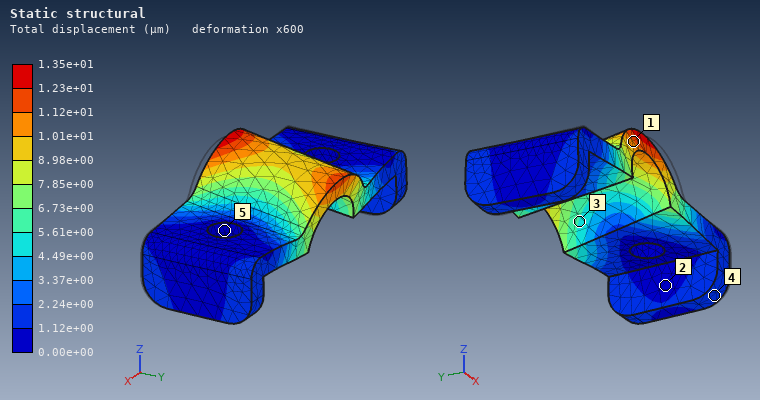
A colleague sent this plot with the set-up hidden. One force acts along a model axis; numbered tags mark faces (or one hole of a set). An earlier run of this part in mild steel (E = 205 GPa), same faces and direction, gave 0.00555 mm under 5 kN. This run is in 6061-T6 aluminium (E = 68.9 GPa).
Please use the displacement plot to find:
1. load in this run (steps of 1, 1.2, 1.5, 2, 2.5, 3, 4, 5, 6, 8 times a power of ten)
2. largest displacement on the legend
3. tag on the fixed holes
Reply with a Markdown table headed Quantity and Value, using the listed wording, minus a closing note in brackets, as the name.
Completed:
| Quantity | Value |
|---|---|
| load in this run | 4 kN |
| largest displacement on the legend | 1.35e+01 µm |
| tag on the fixed holes | 5 |
